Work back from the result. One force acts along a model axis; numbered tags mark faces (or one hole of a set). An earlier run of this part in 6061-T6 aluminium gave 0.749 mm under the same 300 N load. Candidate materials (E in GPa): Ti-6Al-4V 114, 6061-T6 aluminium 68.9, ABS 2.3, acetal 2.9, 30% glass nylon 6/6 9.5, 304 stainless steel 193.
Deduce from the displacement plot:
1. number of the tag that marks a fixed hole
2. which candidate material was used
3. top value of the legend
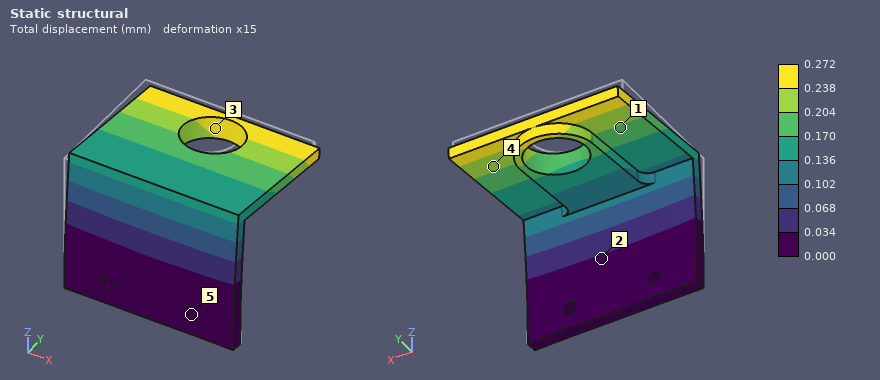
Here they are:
5
304 stainless steel
0.272 mm
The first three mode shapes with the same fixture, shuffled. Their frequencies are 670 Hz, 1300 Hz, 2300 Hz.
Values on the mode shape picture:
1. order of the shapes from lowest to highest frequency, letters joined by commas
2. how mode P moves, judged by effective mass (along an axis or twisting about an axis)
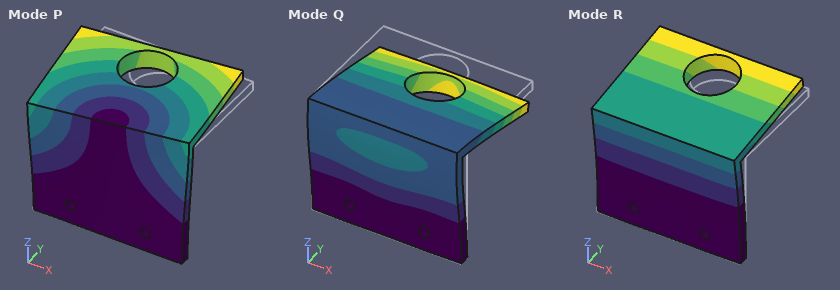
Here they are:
R, P, Q
along X
